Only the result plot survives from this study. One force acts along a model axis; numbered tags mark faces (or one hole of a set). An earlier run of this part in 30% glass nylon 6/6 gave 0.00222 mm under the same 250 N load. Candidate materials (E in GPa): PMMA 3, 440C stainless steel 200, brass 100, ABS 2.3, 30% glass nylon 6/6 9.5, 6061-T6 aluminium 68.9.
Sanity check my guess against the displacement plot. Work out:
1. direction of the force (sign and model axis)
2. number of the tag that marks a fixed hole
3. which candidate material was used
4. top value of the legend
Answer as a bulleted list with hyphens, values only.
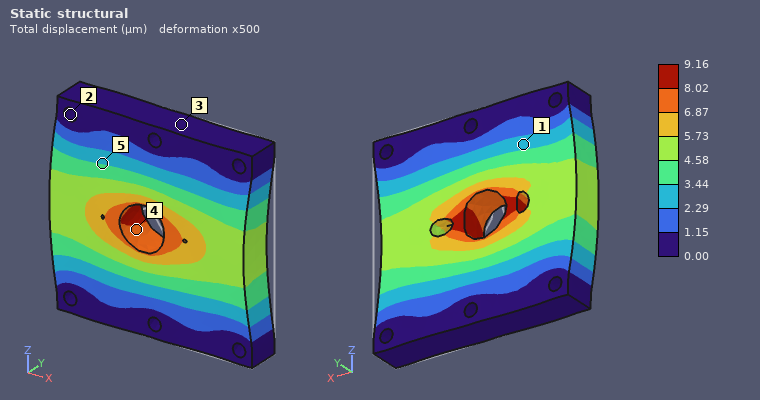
- -X
- 2
- ABS
- 9.16 µm
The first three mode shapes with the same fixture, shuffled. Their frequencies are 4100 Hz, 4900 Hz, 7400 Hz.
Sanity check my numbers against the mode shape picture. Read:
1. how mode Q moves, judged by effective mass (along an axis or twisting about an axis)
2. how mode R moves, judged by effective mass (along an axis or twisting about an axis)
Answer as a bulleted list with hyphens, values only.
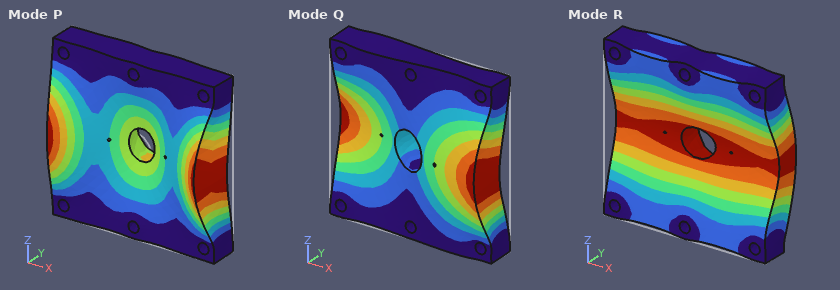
- twisting about Z
- along Y
